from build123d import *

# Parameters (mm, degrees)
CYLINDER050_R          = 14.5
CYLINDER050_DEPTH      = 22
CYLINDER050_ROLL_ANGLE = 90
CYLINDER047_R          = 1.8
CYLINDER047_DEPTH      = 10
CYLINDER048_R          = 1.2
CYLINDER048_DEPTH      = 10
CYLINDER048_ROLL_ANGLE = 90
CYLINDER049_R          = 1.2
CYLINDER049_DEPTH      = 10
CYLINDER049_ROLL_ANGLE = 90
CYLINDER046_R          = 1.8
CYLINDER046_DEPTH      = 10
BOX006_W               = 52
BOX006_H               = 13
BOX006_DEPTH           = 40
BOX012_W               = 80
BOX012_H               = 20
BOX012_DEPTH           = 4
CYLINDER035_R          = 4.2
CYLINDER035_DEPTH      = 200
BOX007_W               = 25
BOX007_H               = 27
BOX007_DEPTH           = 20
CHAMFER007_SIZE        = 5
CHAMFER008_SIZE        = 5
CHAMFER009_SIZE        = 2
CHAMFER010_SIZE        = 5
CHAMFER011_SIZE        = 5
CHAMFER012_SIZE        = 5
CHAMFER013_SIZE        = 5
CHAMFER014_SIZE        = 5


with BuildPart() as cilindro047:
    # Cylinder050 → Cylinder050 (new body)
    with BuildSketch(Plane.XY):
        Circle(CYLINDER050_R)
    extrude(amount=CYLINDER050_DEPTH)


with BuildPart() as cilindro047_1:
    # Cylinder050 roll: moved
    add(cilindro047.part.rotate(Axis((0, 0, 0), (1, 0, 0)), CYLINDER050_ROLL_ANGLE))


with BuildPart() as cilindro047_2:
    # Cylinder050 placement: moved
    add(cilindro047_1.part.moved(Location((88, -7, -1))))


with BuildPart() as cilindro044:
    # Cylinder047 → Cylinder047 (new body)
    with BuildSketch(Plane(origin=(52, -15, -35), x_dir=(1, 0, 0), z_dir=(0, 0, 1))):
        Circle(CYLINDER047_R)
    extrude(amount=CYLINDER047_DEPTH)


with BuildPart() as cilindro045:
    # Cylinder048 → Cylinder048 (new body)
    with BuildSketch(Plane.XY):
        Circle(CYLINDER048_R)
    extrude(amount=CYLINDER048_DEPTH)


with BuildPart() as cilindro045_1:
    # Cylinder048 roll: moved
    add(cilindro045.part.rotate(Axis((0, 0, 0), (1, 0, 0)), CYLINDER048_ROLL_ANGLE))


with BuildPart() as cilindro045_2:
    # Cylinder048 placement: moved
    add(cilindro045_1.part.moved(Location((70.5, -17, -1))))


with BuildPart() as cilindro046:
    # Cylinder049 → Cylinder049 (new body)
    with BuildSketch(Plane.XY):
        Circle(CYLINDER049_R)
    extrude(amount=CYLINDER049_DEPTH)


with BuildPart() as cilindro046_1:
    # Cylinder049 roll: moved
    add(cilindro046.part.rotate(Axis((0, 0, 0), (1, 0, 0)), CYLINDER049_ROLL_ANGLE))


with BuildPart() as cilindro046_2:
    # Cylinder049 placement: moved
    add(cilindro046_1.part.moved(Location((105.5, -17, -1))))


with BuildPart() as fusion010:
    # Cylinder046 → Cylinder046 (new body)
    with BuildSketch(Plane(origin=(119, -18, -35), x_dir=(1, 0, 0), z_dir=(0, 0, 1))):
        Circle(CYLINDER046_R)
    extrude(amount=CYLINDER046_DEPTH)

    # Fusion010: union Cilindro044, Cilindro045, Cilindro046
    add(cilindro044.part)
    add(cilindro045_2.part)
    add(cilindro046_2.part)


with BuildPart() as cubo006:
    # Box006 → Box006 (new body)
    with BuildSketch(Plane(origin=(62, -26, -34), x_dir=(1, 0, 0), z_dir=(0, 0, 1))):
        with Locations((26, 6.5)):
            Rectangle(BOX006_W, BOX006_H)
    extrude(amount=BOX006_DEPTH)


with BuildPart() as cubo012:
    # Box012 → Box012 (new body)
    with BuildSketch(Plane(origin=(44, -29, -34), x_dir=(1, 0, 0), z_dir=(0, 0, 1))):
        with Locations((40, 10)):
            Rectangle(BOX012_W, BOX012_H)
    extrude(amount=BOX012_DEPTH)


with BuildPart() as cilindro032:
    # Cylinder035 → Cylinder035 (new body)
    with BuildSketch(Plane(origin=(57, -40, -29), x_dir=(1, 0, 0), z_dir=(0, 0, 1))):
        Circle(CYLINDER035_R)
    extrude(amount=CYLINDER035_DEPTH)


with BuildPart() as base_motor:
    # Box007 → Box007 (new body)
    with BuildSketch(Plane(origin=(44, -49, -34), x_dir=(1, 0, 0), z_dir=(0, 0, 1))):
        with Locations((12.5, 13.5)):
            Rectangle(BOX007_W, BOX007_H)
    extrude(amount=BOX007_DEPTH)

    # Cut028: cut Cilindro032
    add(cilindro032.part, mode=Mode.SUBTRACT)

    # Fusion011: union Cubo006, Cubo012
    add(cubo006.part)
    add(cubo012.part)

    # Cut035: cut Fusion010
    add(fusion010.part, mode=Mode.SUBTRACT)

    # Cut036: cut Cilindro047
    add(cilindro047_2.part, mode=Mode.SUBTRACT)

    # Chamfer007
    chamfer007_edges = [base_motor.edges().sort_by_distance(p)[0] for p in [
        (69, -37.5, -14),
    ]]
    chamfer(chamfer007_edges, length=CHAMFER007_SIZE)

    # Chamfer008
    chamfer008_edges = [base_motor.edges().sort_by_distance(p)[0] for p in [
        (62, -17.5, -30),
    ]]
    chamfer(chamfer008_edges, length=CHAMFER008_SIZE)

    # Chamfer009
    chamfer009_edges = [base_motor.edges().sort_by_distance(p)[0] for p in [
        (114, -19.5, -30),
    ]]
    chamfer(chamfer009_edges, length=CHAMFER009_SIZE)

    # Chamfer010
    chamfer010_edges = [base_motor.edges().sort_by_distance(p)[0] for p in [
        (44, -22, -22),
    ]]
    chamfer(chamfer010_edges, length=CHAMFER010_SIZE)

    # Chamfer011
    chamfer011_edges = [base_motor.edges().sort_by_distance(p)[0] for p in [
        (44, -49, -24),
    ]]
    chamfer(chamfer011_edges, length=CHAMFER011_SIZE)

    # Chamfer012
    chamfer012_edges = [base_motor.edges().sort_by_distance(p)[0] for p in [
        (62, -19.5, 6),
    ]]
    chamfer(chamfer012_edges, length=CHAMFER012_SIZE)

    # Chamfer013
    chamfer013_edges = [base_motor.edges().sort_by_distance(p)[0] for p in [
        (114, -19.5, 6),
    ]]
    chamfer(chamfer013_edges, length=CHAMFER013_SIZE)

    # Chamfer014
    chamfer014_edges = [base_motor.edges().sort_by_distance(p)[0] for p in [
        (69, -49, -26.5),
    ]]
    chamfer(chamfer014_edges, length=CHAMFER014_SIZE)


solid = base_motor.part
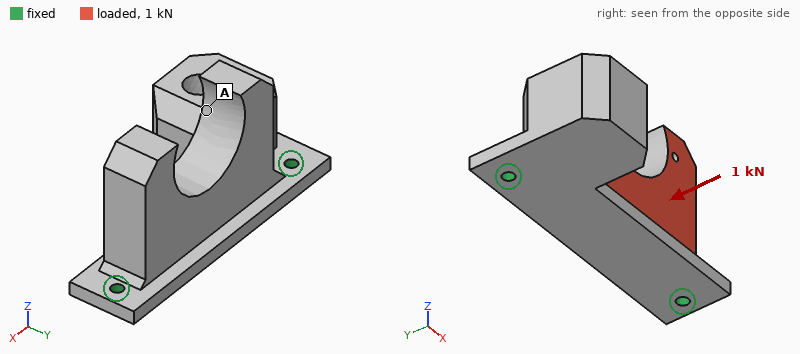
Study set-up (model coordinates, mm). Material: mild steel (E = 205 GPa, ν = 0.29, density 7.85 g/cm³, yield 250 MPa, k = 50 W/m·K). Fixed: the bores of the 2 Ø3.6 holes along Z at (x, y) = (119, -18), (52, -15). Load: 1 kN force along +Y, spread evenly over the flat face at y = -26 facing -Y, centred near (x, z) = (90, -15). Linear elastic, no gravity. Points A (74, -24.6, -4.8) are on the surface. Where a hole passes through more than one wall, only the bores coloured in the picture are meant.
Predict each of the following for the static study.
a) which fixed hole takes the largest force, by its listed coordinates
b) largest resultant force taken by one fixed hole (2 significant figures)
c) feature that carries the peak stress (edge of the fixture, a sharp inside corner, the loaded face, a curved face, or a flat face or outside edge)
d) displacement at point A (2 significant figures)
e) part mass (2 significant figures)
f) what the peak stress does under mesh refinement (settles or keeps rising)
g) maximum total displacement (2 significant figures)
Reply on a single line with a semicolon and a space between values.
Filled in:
(119, -18); 600 N; edge of the fixture; 53 µm; 270 g; keeps rising; 73 µm
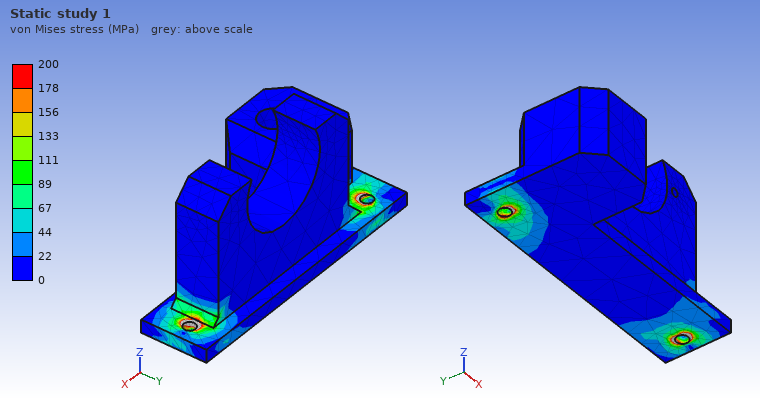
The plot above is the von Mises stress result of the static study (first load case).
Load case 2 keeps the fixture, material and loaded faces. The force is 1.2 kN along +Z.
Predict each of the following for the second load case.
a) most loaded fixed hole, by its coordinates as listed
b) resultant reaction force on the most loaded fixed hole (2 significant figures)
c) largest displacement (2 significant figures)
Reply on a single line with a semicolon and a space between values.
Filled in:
(119, -18); 810 N; 43 µm
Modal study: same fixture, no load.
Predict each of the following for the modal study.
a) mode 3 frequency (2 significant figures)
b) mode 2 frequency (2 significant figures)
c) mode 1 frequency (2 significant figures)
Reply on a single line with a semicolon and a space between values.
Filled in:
6300 Hz; 5000 Hz; 1600 Hz
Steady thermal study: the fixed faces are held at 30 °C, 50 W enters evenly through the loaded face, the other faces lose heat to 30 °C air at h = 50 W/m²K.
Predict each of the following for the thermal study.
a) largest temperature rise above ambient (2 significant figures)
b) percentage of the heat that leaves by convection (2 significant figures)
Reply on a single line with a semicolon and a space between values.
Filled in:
71 K; 38 %
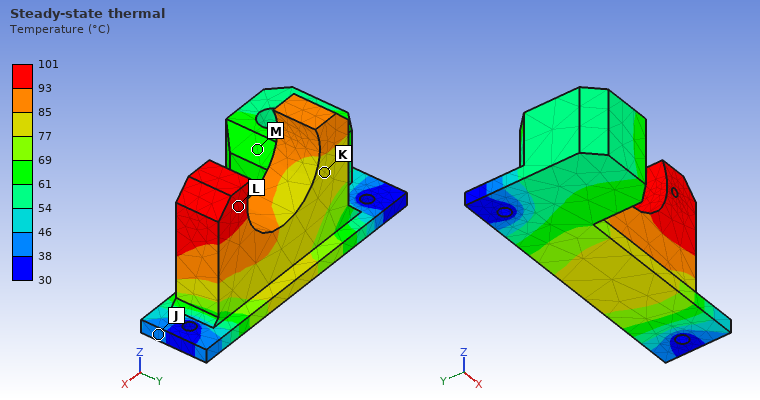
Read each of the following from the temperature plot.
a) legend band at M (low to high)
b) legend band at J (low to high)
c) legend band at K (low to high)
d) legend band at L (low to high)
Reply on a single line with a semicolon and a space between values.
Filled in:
61 to 69 °C; 38 to 46 °C; 77 to 85 °C; 93 to 101 °C
